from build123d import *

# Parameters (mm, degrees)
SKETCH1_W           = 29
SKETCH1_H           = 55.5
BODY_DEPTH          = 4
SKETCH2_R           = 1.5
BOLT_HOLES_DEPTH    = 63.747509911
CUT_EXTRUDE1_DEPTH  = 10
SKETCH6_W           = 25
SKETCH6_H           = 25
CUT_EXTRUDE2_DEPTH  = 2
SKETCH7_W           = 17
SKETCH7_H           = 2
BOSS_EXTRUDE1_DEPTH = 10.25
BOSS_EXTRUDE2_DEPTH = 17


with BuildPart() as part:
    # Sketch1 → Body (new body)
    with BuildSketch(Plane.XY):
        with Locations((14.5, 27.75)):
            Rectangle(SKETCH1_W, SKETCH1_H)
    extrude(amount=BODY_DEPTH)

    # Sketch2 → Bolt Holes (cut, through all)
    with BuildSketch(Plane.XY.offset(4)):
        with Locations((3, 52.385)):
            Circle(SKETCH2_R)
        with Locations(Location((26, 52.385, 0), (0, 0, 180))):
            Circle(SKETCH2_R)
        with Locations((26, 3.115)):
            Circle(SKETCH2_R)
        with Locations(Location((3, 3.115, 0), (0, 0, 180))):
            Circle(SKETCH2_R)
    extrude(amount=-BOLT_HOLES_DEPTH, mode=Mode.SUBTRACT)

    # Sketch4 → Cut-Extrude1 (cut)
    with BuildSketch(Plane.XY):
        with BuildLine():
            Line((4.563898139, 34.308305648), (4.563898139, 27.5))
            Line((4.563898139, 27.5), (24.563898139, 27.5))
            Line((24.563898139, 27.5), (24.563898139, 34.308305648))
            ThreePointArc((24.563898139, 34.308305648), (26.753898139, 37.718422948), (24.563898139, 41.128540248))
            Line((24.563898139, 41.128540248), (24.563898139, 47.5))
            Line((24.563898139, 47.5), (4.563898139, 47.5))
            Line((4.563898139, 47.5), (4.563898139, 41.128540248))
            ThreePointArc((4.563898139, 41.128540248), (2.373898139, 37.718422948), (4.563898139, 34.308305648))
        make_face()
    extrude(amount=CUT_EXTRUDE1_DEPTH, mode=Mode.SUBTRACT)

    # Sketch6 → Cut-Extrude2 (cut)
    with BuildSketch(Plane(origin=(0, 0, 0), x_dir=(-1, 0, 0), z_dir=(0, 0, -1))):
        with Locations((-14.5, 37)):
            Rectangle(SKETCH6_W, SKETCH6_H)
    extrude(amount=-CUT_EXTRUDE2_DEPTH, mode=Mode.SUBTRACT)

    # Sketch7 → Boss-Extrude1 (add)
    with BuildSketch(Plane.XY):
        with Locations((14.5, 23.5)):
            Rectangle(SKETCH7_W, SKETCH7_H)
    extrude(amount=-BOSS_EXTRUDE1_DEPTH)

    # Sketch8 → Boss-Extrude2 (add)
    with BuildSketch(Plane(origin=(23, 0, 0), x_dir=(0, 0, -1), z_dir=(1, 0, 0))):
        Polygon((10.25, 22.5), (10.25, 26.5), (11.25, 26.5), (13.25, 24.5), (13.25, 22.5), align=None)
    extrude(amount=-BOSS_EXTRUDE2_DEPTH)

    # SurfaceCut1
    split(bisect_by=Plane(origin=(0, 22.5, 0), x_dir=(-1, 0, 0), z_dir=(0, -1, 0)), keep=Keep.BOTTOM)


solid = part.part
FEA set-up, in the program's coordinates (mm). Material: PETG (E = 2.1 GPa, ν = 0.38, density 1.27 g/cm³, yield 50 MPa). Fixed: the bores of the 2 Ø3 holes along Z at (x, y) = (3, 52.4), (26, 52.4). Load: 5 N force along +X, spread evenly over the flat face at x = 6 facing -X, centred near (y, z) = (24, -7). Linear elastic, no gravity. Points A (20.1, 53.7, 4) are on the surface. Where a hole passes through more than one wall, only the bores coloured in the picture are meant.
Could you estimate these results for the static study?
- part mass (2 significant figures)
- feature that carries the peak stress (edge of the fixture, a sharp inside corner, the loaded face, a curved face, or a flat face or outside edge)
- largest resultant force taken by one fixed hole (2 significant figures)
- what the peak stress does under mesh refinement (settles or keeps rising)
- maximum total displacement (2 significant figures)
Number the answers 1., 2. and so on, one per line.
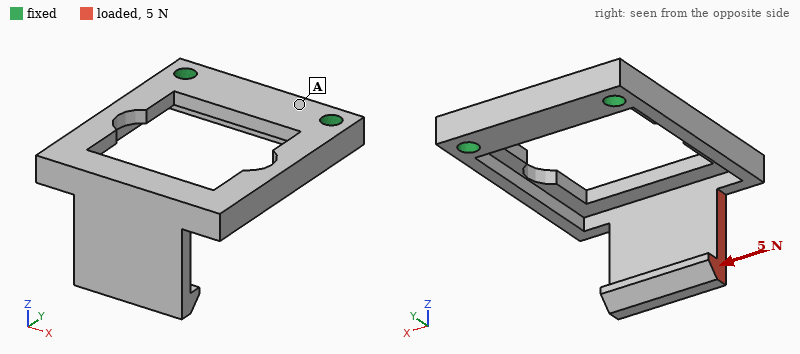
1. 2.8 g
2. a sharp inside corner
3. 5.2 N
4. keeps rising
5. 0.51 mm
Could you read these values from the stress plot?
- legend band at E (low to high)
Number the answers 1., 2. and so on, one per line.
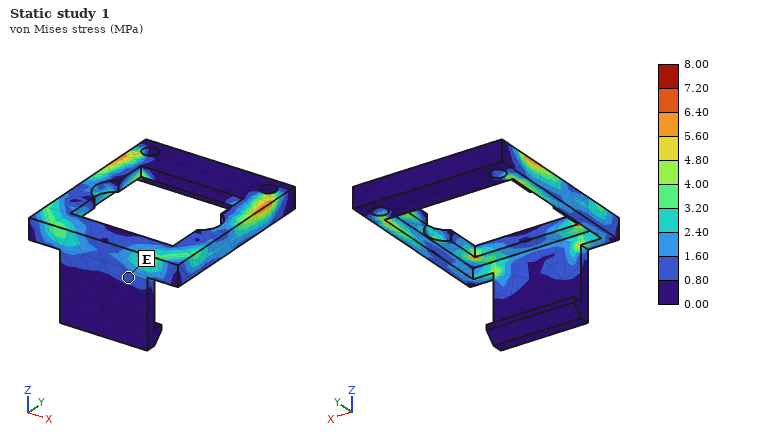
1. 0.80 to 1.60 MPa
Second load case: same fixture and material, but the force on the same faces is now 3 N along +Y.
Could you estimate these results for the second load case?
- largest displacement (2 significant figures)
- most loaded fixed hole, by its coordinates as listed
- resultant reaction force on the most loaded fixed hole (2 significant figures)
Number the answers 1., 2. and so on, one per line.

1. 0.48 mm
2. (3, 52.4)
3. 2.5 N
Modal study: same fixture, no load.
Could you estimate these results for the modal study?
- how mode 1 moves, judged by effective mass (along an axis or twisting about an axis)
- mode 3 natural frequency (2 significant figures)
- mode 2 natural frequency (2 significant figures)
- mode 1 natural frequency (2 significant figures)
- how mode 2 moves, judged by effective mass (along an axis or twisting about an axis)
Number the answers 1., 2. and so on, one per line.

1. along Z
2. 910 Hz
3. 580 Hz
4. 380 Hz
5. along X
